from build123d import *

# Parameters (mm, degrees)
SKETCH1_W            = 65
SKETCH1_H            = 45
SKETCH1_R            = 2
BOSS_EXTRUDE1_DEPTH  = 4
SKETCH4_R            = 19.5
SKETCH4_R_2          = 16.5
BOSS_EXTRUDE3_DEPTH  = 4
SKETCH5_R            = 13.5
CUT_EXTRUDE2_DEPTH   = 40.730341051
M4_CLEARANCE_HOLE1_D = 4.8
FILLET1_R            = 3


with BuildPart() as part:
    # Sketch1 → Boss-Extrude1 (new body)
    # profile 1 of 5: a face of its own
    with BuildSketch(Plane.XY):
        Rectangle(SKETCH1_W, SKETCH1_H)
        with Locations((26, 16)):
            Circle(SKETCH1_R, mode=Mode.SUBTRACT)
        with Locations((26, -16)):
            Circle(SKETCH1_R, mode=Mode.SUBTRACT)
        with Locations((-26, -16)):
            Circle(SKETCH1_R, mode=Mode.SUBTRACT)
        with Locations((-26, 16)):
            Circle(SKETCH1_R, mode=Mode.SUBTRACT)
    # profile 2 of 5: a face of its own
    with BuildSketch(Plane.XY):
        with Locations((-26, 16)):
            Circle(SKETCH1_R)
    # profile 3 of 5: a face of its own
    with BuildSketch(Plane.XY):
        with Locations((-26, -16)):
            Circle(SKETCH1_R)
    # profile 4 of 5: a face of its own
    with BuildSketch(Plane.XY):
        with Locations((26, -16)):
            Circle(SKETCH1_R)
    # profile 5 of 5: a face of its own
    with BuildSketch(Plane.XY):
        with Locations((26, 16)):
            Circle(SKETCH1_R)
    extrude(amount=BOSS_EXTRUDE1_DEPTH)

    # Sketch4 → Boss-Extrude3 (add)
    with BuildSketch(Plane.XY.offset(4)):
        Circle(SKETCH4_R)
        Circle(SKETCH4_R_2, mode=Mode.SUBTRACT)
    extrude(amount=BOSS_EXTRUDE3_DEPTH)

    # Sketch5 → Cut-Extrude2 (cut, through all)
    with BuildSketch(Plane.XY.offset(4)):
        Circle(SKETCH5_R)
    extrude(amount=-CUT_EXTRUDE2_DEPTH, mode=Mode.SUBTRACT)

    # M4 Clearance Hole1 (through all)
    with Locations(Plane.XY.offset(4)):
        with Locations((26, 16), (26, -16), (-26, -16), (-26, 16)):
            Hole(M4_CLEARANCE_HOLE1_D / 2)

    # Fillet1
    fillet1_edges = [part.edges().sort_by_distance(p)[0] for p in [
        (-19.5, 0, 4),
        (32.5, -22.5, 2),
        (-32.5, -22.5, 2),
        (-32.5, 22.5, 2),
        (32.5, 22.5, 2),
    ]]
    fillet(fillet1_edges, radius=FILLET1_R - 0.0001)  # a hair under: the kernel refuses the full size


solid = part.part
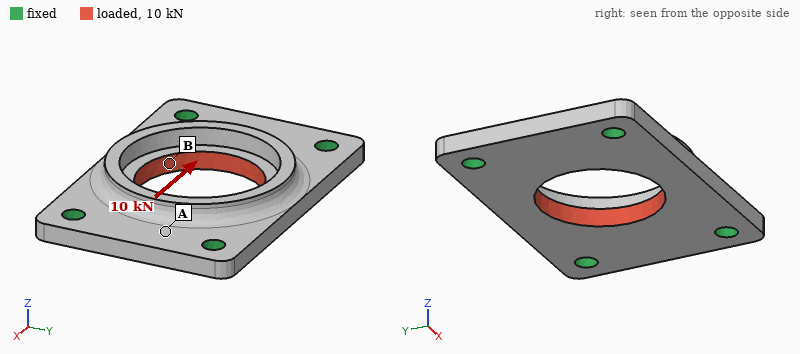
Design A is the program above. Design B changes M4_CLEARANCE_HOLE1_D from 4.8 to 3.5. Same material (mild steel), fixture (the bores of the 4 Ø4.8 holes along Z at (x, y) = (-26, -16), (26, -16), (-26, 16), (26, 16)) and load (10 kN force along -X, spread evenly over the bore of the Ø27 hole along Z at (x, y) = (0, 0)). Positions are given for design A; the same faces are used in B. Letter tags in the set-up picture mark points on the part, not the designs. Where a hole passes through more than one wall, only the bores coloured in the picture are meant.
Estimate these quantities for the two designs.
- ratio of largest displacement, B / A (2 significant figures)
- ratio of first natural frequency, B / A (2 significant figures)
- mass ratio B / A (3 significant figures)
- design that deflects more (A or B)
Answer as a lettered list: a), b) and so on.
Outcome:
a) 1.1
b) 0.92
c) 1.01
d) B
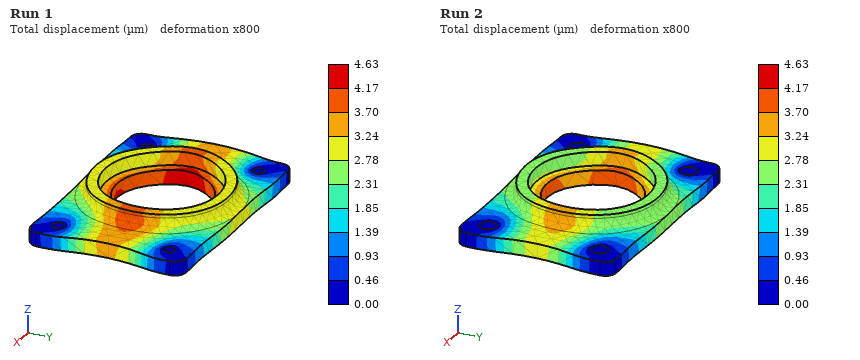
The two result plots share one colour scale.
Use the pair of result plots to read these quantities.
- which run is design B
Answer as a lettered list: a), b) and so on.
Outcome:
a) Run 1
